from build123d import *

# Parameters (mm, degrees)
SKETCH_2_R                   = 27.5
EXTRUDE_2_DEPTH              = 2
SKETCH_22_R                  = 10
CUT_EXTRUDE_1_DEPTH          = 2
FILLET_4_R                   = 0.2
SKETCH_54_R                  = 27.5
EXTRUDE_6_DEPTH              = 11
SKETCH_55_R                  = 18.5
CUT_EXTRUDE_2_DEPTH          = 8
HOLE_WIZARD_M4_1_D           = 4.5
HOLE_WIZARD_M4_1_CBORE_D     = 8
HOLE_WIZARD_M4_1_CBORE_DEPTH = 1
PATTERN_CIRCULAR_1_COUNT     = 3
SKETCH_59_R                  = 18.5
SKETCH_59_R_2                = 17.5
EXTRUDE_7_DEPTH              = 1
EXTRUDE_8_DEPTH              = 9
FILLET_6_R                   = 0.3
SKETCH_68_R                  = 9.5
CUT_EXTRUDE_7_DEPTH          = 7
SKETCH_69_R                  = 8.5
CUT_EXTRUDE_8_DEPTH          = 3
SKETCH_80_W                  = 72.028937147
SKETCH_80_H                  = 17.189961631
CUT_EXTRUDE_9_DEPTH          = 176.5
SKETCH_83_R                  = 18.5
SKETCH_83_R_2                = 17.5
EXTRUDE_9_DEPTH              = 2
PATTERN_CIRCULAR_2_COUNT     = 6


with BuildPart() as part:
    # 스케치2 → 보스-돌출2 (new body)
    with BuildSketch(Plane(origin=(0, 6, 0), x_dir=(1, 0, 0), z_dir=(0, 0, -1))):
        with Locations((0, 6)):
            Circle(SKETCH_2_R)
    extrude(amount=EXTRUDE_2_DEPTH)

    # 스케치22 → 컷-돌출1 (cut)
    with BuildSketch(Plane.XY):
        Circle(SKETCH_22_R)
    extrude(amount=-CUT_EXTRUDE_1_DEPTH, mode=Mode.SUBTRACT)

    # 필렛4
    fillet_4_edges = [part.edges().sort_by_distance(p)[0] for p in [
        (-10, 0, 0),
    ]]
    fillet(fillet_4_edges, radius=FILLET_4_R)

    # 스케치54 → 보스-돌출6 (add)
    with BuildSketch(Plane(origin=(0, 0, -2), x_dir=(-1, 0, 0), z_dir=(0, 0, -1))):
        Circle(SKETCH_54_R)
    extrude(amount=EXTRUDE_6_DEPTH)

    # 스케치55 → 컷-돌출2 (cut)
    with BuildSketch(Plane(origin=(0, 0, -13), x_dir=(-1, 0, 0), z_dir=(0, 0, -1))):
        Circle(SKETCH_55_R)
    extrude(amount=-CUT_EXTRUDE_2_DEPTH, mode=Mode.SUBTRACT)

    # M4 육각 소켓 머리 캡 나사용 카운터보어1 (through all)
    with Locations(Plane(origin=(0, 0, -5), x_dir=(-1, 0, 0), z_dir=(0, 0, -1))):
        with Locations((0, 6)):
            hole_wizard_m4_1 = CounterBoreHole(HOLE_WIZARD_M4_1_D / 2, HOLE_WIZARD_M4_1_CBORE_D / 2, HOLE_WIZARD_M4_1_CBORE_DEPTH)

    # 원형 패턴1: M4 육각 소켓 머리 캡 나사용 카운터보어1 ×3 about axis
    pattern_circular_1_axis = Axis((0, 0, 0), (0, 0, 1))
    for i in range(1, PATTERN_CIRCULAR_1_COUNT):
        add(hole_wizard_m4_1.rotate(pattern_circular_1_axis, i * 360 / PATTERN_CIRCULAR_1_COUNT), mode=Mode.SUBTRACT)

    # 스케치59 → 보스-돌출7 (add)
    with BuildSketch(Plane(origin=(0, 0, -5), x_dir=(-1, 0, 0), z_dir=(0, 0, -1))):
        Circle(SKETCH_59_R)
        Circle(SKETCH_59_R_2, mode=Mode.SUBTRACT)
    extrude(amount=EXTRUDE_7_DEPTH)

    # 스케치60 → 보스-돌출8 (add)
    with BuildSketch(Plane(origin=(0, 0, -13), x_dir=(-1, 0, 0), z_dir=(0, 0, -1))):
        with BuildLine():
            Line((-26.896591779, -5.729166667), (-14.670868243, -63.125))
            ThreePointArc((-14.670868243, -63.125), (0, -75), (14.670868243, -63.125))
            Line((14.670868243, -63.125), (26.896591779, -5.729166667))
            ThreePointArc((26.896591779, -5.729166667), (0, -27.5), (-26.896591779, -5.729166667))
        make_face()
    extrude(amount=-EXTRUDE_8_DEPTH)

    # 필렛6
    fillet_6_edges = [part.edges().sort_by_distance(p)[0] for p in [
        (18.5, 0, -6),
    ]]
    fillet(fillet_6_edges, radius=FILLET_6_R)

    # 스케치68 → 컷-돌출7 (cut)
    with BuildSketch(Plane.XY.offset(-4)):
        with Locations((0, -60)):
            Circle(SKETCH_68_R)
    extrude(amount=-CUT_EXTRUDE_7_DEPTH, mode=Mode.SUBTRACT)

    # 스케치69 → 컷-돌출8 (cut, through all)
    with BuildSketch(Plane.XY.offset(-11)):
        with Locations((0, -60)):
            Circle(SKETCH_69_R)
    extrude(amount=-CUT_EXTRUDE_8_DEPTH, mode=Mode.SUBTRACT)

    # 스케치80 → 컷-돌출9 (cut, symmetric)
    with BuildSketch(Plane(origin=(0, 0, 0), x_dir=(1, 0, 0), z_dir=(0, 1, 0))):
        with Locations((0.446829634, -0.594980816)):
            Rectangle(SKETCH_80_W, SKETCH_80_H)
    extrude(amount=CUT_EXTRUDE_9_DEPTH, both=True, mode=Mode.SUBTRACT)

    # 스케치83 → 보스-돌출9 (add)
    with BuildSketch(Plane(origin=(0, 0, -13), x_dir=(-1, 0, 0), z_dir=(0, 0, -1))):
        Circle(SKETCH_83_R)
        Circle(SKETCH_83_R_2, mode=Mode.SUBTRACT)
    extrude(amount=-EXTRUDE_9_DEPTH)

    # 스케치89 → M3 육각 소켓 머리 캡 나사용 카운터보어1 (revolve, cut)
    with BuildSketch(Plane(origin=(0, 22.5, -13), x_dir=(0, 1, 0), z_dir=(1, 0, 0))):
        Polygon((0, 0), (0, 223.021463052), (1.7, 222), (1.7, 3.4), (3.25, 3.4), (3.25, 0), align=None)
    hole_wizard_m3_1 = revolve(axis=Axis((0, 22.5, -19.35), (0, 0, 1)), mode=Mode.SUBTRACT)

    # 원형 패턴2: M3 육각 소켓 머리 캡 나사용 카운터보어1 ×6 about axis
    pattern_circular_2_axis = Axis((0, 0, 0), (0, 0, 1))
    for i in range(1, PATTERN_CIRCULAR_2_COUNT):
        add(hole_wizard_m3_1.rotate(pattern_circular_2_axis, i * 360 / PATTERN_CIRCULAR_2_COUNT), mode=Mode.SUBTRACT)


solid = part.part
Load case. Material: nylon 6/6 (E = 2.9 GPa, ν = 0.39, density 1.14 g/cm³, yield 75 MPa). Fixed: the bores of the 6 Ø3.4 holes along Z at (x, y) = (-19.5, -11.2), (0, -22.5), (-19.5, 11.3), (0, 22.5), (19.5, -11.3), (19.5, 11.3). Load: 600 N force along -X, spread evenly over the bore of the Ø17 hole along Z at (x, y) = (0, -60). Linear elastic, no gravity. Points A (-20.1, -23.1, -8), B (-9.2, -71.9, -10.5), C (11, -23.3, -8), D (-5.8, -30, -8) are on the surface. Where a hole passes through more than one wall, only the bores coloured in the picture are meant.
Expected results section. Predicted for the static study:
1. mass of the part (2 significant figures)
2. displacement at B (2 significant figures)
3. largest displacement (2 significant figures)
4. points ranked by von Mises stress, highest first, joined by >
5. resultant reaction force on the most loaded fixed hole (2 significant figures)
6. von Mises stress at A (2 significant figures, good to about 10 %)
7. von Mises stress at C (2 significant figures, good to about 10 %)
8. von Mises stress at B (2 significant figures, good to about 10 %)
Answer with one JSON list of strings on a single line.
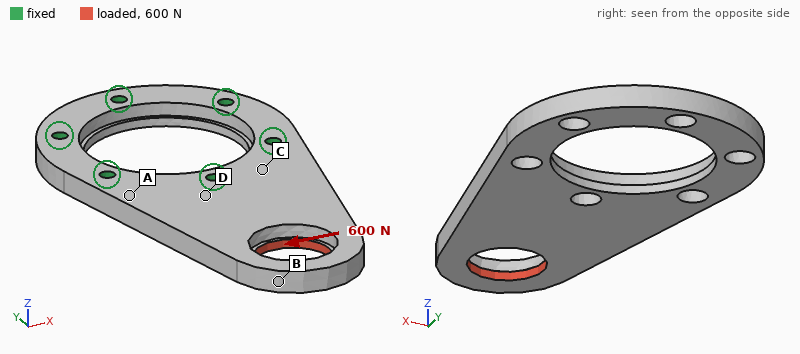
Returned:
["15 g", "0.75 mm", "0.81 mm", "A > B > C > D", "540 N", "17 MPa", "6.7 MPa", "12 MPa"]
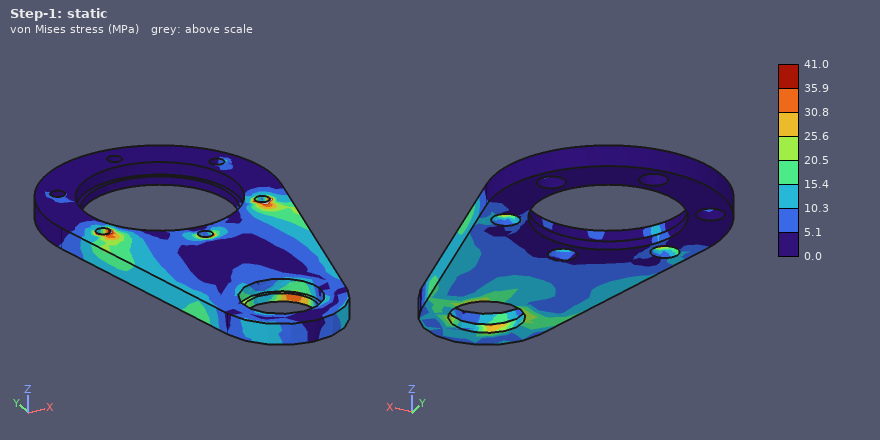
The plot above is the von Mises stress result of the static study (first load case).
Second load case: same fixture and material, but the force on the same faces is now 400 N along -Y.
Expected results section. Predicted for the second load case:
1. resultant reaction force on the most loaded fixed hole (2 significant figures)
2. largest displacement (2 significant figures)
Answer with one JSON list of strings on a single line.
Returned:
["140 N", "1.2 mm"]
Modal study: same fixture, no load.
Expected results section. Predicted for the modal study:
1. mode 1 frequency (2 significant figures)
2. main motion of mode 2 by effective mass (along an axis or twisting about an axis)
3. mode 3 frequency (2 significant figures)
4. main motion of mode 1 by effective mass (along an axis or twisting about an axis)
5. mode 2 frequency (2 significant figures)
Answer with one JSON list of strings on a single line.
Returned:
["520 Hz", "twisting about Y", "2100 Hz", "along Z", "1400 Hz"]
